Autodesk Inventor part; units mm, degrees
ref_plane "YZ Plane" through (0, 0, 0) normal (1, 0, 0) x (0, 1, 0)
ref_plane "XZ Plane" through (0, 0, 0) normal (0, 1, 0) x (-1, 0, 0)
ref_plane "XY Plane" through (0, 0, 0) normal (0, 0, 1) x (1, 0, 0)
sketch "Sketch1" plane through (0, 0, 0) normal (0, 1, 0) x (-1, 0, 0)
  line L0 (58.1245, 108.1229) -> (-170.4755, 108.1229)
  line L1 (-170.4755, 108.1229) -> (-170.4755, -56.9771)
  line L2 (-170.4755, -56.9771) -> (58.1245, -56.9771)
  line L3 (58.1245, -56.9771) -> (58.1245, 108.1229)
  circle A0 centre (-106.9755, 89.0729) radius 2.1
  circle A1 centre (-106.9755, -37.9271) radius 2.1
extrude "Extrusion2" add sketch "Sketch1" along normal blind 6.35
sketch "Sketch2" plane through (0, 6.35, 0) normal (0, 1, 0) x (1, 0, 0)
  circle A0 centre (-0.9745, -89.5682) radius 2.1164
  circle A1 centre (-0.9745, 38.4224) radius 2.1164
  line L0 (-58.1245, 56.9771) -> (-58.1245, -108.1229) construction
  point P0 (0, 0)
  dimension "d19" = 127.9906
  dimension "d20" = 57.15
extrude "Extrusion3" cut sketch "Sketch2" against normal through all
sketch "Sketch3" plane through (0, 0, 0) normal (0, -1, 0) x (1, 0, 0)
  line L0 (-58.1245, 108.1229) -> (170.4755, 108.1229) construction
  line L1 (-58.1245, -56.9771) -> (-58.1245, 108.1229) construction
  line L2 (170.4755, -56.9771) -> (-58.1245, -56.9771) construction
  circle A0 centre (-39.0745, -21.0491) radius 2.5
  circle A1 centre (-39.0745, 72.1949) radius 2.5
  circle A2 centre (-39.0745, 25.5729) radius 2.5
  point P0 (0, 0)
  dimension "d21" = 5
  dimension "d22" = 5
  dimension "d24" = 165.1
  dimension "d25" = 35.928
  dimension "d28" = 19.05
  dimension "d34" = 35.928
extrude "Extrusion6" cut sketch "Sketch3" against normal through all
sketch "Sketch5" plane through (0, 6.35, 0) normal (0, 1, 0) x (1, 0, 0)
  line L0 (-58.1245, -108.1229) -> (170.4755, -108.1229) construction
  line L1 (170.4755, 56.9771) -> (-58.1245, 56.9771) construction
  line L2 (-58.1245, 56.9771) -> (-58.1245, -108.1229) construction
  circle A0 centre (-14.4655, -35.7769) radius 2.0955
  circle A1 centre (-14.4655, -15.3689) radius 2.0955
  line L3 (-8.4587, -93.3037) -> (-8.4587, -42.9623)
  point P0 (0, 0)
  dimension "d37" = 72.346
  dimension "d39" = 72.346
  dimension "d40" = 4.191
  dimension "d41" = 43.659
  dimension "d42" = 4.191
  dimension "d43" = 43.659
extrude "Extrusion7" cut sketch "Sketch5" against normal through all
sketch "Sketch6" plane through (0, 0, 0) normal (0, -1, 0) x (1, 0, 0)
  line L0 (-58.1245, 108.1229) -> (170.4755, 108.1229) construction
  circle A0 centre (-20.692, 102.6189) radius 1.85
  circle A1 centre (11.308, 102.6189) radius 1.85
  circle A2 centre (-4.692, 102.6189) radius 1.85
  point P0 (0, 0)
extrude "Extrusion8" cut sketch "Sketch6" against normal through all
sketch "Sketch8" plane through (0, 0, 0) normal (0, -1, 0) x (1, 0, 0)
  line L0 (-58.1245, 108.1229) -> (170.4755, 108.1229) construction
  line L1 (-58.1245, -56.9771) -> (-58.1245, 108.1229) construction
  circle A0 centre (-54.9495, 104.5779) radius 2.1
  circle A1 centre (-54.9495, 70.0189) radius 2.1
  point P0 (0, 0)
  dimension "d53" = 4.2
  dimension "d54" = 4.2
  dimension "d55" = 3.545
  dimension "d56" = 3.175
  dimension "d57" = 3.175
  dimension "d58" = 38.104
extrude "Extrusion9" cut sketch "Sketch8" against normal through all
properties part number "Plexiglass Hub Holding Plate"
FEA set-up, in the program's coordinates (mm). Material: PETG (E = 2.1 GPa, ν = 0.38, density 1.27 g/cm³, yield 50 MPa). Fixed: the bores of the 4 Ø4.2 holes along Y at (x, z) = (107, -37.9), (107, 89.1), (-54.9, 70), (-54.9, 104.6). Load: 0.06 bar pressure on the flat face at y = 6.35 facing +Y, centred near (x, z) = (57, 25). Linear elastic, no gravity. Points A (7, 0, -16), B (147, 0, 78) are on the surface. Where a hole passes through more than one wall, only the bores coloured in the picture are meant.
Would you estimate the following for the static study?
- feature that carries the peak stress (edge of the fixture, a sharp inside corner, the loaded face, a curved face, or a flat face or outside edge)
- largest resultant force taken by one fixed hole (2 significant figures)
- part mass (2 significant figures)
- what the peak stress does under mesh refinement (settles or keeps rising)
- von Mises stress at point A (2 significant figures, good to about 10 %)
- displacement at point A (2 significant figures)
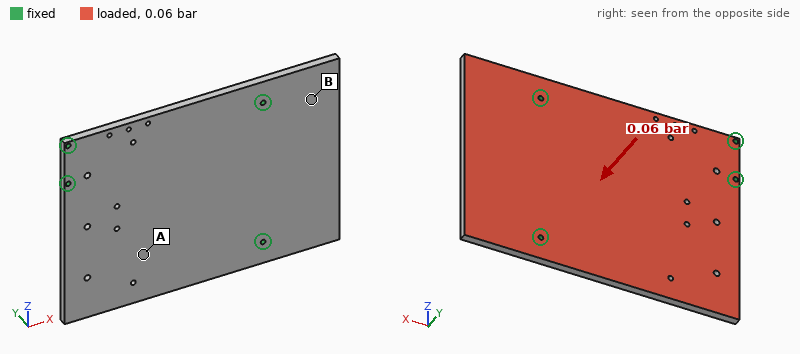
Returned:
edge of the fixture
92 N
300 g
keeps rising
2.0 MPa
1.4 mm
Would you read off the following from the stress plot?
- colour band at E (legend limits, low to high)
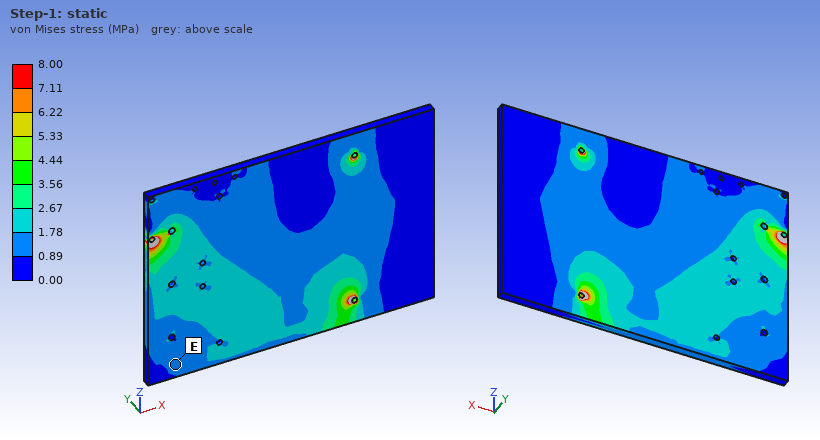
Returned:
0.89 to 1.78 MPa
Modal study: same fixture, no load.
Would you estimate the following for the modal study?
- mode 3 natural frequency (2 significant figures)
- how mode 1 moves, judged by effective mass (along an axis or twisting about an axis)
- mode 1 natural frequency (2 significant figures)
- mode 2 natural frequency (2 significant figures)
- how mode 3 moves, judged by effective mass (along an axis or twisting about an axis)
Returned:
270 Hz
along Y
110 Hz
220 Hz
along Y
